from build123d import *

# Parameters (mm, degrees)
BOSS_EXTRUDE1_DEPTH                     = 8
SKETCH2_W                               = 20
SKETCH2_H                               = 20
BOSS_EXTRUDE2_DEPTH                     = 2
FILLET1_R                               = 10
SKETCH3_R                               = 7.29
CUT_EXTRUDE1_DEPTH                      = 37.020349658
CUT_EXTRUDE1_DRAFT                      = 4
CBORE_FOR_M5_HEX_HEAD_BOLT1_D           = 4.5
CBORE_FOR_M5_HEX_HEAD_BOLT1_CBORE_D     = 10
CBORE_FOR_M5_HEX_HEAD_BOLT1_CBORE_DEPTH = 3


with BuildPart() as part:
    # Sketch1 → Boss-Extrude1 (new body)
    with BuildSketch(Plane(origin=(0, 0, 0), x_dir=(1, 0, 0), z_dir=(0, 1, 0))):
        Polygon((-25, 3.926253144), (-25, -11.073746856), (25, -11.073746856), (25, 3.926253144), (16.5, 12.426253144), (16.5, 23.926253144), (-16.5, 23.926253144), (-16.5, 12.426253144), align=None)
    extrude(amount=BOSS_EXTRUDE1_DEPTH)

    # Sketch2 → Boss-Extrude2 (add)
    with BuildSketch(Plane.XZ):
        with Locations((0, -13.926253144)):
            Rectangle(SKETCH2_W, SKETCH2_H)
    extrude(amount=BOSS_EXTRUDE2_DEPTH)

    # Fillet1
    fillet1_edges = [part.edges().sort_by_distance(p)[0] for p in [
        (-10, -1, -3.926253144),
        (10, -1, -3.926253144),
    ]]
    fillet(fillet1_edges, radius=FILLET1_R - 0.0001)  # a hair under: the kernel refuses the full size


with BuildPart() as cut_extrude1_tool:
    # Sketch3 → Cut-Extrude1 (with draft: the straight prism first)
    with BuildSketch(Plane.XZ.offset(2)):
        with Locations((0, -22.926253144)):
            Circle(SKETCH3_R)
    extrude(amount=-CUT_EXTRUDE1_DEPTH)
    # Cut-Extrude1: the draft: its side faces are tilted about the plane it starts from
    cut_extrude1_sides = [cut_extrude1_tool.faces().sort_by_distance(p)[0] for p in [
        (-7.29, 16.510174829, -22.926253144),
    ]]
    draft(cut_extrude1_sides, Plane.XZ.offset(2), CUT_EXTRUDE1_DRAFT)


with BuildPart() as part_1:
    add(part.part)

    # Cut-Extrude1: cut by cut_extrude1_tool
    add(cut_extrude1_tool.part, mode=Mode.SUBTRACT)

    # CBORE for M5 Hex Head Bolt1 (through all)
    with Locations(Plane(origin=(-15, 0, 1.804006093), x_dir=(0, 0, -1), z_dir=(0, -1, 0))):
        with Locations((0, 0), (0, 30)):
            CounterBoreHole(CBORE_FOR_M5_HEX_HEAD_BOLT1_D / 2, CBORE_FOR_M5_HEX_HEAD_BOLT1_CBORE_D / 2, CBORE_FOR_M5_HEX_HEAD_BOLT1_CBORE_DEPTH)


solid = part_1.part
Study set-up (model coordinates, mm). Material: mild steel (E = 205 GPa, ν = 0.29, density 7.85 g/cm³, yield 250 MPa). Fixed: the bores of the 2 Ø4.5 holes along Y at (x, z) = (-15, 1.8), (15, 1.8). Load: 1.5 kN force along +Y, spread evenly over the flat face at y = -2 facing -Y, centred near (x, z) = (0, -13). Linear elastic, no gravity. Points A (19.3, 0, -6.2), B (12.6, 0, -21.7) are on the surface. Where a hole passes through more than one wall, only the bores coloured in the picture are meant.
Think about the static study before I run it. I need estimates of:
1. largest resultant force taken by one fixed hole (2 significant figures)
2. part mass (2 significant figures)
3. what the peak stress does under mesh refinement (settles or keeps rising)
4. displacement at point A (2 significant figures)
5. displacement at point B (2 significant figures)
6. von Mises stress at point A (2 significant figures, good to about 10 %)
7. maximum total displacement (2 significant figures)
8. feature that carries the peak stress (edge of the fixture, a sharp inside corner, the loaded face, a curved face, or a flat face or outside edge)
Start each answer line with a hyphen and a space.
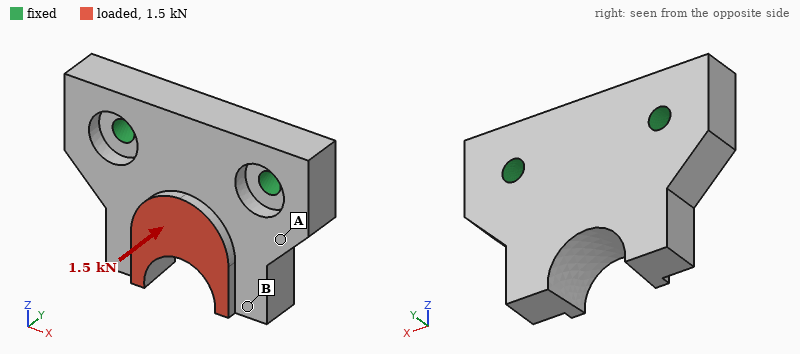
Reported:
- 800 N
- 85 g
- keeps rising
- 6.1 µm
- 23 µm
- 39 MPa
- 27 µm
- edge of the fixture
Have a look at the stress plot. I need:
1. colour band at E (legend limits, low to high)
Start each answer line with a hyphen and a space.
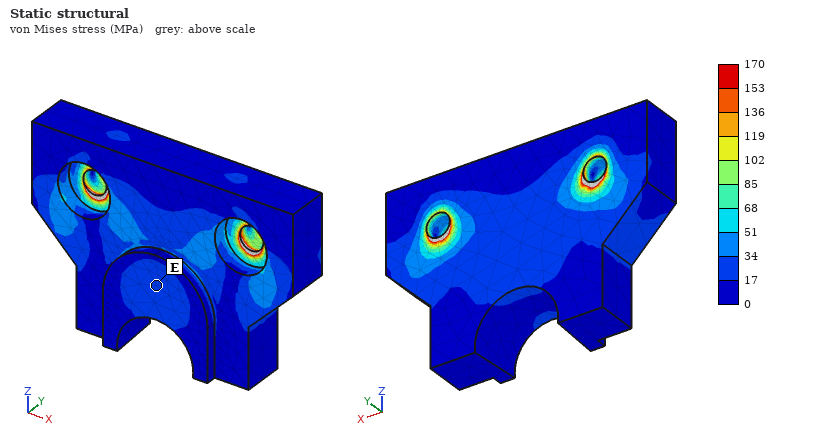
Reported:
- 17 to 34 MPa
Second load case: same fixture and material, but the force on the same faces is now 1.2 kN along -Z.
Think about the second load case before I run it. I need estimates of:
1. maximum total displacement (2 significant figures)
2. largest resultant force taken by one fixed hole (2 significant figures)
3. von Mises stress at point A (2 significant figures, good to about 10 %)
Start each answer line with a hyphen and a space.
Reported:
- 13 µm
- 620 N
- 19 MPa
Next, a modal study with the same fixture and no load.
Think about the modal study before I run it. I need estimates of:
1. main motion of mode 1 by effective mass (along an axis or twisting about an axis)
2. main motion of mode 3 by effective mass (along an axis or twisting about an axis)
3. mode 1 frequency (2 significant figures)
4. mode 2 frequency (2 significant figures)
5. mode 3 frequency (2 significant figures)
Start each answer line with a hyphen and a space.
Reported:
- along Y
- along Y
- 7600 Hz
- 16 kHz
- 25 kHz
